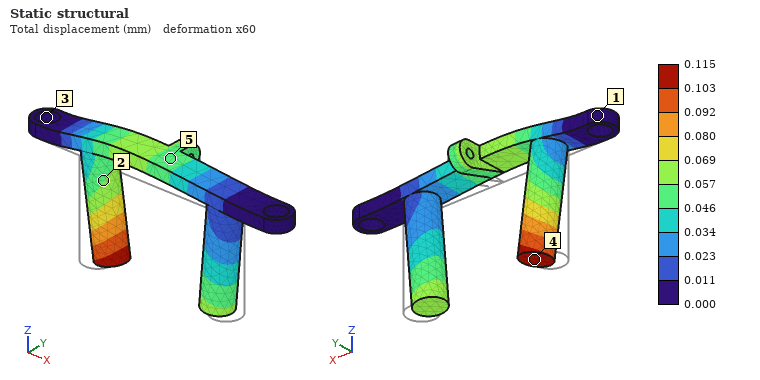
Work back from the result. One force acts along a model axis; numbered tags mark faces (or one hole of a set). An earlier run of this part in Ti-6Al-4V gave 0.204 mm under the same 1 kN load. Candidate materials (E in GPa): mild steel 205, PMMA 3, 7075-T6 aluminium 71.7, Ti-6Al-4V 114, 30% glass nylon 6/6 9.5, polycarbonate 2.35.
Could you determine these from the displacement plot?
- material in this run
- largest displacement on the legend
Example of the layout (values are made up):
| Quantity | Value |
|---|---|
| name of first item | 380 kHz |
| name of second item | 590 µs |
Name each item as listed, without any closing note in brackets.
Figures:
| Quantity | Value |
|---|---|
| material in this run | mild steel |
| largest displacement on the legend | 0.115 mm |
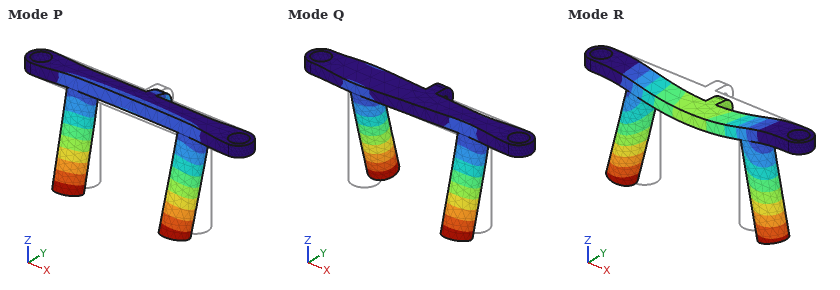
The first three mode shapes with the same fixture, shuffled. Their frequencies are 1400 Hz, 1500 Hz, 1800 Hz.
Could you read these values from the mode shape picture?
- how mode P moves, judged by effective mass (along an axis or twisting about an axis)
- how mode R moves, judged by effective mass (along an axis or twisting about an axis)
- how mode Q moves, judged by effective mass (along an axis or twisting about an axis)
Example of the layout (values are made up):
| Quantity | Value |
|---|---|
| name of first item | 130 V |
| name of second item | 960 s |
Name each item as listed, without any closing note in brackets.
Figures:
| Quantity | Value |
|---|---|
| how mode P moves, judged by effective mass | along Y |
| how mode R moves, judged by effective mass | along Z |
| how mode Q moves, judged by effective mass | twisting about Z |
